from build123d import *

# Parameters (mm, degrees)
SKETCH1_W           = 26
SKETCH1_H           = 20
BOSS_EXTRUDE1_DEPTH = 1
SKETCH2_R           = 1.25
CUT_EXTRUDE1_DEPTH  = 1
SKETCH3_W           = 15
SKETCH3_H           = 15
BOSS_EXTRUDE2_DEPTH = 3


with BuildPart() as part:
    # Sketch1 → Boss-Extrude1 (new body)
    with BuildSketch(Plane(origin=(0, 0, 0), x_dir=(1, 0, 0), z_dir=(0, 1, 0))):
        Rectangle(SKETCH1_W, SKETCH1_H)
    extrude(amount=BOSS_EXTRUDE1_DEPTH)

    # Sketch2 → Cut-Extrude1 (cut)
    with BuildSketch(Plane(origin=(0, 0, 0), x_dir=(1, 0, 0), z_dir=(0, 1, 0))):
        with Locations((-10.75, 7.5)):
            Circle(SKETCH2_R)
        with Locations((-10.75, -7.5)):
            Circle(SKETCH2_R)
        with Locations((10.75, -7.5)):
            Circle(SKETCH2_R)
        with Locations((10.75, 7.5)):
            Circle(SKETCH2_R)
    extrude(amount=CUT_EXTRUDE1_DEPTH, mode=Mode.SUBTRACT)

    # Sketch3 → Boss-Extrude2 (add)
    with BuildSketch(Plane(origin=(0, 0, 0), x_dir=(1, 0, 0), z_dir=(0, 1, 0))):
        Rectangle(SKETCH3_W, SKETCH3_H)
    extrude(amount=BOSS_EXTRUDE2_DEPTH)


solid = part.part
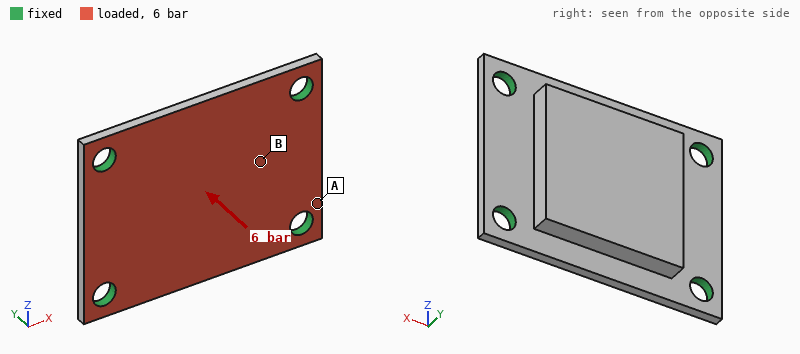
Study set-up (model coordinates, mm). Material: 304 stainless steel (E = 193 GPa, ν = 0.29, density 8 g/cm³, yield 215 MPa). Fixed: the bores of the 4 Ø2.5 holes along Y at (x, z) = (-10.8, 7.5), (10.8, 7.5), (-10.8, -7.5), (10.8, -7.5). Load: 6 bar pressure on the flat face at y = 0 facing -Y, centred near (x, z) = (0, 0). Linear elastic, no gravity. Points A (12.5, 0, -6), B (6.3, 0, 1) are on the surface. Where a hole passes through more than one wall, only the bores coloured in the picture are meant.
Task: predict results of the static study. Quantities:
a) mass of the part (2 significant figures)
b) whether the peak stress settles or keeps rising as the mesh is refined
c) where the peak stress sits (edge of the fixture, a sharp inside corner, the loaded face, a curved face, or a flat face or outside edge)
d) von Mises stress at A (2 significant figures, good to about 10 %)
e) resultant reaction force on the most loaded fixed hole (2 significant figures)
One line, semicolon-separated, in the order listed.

7.6 g; keeps rising; edge of the fixture; 25 MPa; 90 N
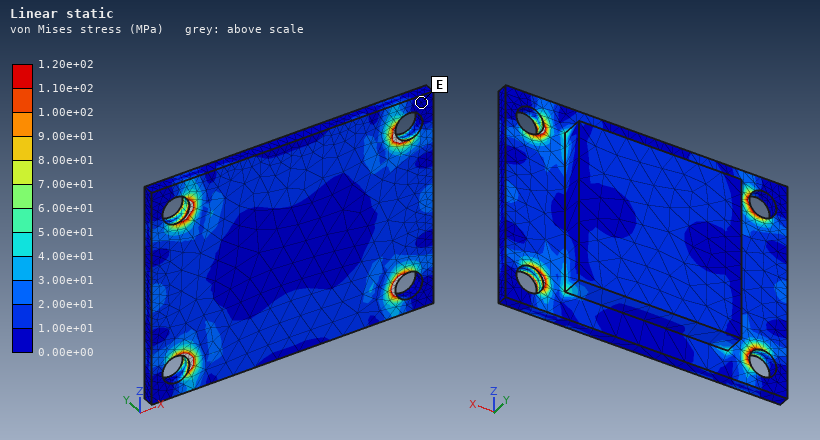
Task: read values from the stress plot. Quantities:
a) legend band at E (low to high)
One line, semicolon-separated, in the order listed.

0.00e+00 to 1.00e+01 MPa
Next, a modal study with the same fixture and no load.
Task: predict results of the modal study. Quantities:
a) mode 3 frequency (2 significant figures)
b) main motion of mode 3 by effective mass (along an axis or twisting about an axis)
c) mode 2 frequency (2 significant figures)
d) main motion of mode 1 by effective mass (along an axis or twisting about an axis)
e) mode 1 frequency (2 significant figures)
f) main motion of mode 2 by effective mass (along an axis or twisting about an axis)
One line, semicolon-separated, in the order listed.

31 kHz; twisting about Z; 23 kHz; along Y; 16 kHz; twisting about X
